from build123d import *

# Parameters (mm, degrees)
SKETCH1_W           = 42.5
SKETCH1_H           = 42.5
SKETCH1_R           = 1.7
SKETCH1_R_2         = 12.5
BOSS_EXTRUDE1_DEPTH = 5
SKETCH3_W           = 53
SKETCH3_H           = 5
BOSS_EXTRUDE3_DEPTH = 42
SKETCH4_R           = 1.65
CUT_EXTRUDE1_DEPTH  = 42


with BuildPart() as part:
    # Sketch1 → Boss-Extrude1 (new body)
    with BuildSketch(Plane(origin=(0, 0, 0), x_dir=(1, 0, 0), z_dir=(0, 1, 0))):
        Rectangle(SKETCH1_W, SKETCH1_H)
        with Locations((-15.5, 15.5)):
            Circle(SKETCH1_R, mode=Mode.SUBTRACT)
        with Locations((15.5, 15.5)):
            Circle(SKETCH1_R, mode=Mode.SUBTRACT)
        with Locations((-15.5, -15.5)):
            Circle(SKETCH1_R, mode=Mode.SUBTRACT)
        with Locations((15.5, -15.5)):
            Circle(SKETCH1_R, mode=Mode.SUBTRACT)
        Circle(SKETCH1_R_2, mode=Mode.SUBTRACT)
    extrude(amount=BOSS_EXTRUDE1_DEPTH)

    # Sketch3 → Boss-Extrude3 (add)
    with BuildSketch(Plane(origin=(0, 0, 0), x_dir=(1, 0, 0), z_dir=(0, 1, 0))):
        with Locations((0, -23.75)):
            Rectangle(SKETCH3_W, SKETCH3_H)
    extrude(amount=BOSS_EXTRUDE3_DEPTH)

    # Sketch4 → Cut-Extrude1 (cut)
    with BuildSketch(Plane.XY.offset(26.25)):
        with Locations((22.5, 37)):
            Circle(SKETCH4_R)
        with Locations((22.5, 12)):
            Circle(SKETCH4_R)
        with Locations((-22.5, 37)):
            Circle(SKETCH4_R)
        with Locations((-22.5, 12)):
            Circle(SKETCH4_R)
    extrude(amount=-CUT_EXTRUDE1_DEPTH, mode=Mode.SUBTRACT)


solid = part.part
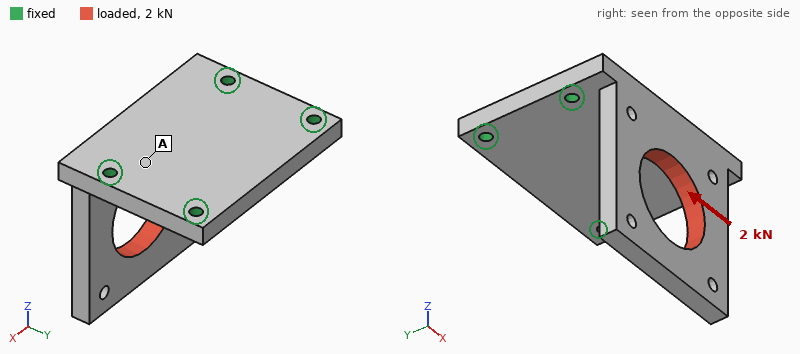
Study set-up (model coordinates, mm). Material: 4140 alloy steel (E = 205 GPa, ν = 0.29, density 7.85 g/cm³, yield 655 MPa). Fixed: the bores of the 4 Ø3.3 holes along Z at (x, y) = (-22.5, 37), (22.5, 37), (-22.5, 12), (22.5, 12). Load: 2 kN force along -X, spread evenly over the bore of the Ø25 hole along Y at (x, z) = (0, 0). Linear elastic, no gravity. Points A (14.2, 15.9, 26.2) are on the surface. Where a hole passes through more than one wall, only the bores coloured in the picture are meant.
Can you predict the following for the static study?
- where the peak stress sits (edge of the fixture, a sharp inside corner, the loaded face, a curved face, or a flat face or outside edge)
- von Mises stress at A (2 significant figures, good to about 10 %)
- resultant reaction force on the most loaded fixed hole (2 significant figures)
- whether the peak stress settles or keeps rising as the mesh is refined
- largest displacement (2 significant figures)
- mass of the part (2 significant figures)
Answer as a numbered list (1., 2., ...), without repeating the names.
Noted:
1. edge of the fixture
2. 16 MPa
3. 1.5 kN
4. keeps rising
5. 46 µm
6. 140 g
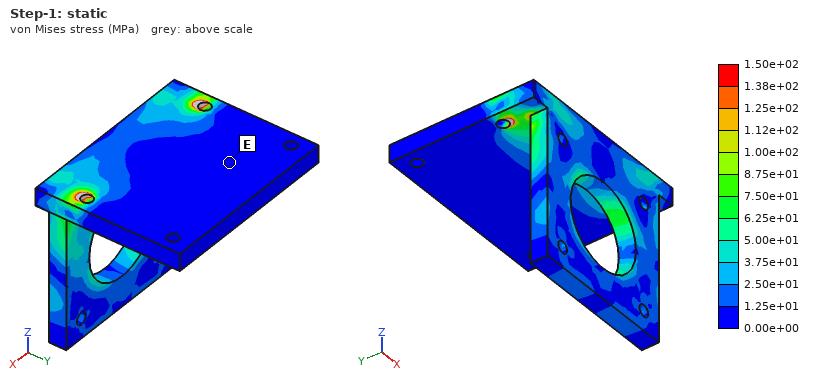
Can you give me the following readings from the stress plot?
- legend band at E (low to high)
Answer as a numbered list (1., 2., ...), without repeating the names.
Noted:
1. 0.00e+00 to 1.25e+01 MPa
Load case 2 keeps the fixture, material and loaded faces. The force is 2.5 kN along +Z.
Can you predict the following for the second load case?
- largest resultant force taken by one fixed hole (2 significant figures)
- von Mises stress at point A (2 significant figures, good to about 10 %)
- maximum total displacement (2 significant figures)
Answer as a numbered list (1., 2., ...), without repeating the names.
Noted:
1. 1.4 kN
2. 38 MPa
3. 71 µm
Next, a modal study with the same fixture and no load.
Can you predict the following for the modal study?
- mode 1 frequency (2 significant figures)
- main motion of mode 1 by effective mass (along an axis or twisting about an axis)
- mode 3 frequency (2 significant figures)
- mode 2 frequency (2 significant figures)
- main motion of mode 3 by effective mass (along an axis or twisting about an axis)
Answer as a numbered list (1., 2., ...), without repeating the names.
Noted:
1. 1500 Hz
2. along Y
3. 5600 Hz
4. 3800 Hz
5. along X
